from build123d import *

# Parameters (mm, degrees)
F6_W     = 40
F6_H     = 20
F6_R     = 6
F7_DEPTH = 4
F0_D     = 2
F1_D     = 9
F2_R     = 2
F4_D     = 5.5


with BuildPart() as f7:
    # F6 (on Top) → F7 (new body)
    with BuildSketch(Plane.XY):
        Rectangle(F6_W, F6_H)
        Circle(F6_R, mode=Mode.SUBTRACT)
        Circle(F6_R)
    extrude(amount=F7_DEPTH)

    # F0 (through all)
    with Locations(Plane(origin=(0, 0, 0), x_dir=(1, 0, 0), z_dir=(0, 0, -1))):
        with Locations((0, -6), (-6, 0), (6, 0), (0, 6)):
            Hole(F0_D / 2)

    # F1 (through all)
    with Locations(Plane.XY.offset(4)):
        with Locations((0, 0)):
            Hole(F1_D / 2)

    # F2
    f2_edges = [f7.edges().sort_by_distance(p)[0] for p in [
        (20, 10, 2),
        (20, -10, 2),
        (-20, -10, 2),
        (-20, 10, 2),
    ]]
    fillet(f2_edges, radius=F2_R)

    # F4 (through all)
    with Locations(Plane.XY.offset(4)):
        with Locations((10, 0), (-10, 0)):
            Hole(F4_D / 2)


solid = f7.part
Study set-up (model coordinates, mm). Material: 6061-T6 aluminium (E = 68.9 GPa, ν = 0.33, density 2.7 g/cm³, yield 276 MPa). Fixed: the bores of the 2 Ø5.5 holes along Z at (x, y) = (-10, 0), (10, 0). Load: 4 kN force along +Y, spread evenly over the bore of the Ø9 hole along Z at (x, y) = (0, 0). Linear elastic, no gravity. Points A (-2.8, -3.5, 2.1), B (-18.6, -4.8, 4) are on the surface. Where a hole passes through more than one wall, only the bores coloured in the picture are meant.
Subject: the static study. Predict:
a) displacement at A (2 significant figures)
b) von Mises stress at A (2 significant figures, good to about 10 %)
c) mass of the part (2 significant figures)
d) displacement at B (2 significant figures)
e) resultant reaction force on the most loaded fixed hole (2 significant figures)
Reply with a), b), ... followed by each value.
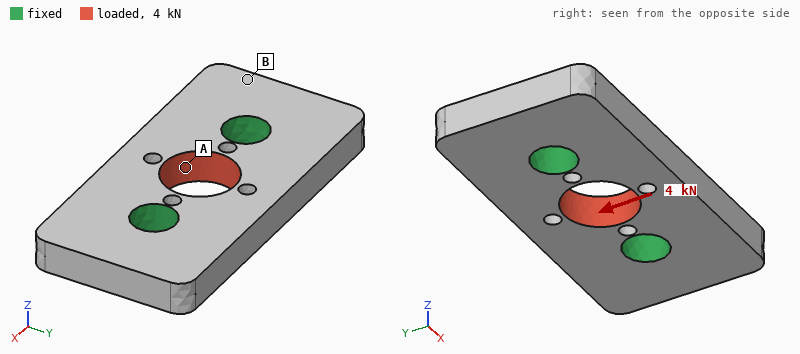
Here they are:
a) 9.7 µm
b) 60 MPa
c) 7.3 g
d) 2.4 µm
e) 2.0 kN
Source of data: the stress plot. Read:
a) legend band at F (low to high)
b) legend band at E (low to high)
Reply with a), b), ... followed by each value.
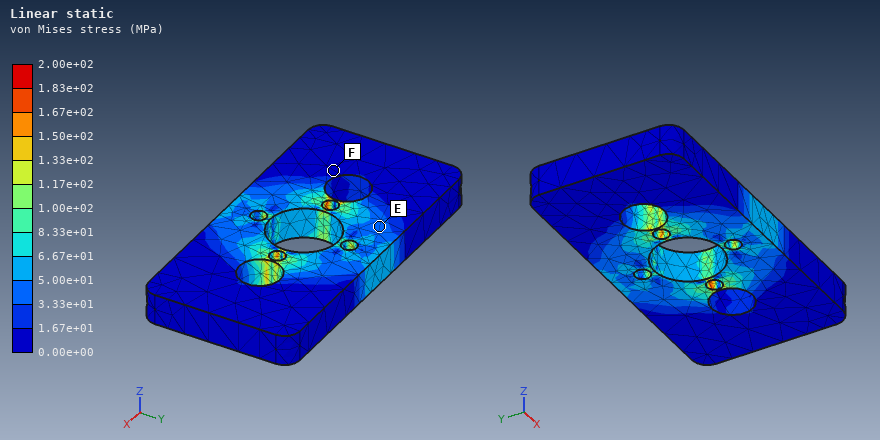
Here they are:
a) 0.00e+00 to 1.67e+01 MPa
b) 3.33e+01 to 5.00e+01 MPa
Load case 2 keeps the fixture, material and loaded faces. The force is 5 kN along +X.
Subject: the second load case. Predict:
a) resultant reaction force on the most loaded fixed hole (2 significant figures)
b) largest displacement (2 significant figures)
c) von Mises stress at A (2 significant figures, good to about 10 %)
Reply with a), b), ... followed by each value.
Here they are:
a) 2.5 kN
b) 7.4 µm
c) 79 MPa
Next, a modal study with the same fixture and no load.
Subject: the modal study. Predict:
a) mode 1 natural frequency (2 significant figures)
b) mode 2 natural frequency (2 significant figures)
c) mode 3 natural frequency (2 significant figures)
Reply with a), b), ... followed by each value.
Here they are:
a) 31 kHz
b) 32 kHz
c) 32 kHz
